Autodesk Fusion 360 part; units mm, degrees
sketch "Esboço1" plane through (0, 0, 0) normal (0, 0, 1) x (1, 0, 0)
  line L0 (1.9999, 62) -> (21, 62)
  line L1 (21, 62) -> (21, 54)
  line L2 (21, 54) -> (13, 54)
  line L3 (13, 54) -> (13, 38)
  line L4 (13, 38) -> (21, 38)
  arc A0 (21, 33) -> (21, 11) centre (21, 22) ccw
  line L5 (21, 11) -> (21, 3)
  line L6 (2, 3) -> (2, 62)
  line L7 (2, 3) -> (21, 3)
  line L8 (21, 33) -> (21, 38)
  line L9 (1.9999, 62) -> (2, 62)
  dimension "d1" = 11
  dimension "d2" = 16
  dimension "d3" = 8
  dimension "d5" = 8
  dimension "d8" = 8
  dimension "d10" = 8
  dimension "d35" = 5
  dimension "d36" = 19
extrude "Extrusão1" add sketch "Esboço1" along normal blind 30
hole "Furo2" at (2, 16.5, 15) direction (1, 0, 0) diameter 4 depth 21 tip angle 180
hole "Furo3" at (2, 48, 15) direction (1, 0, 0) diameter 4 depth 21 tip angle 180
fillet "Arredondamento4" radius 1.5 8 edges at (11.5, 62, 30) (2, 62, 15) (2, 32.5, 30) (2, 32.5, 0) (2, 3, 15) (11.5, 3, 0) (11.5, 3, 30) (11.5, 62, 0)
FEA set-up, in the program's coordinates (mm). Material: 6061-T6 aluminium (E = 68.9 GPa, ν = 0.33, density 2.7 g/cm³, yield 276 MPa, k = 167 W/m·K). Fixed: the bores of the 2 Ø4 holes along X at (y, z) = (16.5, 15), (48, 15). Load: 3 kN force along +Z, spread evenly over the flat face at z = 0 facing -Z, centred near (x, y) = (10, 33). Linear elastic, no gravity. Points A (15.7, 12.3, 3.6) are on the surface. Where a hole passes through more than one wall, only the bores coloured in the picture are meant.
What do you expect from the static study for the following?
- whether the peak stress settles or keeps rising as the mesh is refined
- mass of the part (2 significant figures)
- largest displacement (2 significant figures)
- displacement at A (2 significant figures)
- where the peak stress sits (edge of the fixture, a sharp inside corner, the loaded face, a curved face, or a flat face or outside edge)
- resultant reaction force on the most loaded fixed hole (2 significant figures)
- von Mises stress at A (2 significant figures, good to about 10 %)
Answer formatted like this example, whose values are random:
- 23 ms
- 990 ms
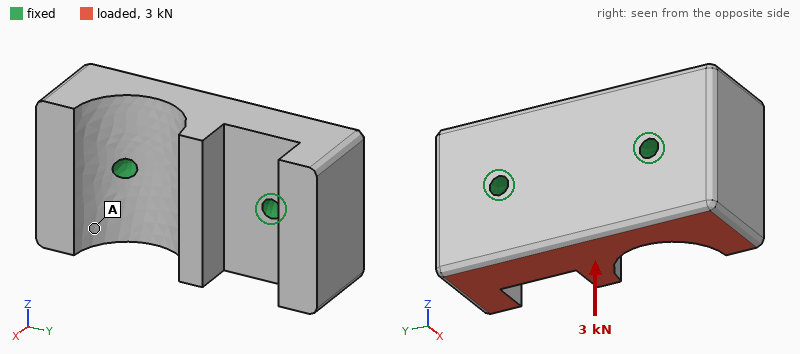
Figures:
- keeps rising
- 64 g
- 5.8 µm
- 3.7 µm
- edge of the fixture
- 1.6 kN
- 5.4 MPa
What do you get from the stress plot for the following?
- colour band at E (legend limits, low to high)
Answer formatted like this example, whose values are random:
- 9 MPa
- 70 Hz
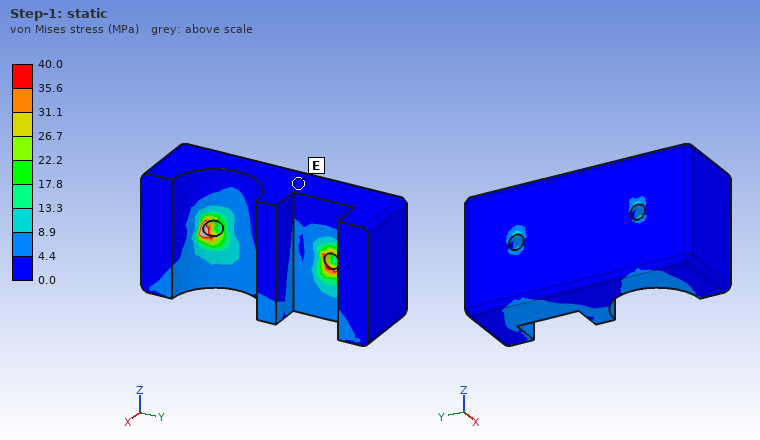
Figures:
- 0.0 to 4.4 MPa
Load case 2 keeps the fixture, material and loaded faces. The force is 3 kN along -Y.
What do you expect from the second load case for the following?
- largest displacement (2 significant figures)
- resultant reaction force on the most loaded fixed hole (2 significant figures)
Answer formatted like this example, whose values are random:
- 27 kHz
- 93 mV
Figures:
- 12 µm
- 2.0 kN
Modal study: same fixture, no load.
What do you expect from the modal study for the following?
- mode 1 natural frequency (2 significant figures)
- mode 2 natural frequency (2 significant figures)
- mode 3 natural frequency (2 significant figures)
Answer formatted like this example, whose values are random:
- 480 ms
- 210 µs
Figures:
- 14 kHz
- 17 kHz
- 17 kHz
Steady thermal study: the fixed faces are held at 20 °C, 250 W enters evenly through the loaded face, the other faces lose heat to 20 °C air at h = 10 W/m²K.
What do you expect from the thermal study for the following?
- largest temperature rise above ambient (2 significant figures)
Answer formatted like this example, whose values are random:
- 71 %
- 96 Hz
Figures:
- 48 K
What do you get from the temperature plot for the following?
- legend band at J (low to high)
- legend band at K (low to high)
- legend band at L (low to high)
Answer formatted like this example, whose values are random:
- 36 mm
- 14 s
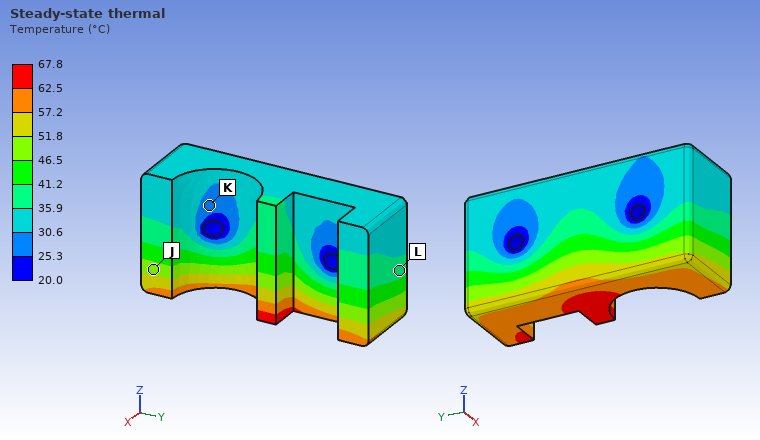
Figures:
- 46.5 to 51.8 °C
- 25.3 to 30.6 °C
- 35.9 to 41.2 °C
